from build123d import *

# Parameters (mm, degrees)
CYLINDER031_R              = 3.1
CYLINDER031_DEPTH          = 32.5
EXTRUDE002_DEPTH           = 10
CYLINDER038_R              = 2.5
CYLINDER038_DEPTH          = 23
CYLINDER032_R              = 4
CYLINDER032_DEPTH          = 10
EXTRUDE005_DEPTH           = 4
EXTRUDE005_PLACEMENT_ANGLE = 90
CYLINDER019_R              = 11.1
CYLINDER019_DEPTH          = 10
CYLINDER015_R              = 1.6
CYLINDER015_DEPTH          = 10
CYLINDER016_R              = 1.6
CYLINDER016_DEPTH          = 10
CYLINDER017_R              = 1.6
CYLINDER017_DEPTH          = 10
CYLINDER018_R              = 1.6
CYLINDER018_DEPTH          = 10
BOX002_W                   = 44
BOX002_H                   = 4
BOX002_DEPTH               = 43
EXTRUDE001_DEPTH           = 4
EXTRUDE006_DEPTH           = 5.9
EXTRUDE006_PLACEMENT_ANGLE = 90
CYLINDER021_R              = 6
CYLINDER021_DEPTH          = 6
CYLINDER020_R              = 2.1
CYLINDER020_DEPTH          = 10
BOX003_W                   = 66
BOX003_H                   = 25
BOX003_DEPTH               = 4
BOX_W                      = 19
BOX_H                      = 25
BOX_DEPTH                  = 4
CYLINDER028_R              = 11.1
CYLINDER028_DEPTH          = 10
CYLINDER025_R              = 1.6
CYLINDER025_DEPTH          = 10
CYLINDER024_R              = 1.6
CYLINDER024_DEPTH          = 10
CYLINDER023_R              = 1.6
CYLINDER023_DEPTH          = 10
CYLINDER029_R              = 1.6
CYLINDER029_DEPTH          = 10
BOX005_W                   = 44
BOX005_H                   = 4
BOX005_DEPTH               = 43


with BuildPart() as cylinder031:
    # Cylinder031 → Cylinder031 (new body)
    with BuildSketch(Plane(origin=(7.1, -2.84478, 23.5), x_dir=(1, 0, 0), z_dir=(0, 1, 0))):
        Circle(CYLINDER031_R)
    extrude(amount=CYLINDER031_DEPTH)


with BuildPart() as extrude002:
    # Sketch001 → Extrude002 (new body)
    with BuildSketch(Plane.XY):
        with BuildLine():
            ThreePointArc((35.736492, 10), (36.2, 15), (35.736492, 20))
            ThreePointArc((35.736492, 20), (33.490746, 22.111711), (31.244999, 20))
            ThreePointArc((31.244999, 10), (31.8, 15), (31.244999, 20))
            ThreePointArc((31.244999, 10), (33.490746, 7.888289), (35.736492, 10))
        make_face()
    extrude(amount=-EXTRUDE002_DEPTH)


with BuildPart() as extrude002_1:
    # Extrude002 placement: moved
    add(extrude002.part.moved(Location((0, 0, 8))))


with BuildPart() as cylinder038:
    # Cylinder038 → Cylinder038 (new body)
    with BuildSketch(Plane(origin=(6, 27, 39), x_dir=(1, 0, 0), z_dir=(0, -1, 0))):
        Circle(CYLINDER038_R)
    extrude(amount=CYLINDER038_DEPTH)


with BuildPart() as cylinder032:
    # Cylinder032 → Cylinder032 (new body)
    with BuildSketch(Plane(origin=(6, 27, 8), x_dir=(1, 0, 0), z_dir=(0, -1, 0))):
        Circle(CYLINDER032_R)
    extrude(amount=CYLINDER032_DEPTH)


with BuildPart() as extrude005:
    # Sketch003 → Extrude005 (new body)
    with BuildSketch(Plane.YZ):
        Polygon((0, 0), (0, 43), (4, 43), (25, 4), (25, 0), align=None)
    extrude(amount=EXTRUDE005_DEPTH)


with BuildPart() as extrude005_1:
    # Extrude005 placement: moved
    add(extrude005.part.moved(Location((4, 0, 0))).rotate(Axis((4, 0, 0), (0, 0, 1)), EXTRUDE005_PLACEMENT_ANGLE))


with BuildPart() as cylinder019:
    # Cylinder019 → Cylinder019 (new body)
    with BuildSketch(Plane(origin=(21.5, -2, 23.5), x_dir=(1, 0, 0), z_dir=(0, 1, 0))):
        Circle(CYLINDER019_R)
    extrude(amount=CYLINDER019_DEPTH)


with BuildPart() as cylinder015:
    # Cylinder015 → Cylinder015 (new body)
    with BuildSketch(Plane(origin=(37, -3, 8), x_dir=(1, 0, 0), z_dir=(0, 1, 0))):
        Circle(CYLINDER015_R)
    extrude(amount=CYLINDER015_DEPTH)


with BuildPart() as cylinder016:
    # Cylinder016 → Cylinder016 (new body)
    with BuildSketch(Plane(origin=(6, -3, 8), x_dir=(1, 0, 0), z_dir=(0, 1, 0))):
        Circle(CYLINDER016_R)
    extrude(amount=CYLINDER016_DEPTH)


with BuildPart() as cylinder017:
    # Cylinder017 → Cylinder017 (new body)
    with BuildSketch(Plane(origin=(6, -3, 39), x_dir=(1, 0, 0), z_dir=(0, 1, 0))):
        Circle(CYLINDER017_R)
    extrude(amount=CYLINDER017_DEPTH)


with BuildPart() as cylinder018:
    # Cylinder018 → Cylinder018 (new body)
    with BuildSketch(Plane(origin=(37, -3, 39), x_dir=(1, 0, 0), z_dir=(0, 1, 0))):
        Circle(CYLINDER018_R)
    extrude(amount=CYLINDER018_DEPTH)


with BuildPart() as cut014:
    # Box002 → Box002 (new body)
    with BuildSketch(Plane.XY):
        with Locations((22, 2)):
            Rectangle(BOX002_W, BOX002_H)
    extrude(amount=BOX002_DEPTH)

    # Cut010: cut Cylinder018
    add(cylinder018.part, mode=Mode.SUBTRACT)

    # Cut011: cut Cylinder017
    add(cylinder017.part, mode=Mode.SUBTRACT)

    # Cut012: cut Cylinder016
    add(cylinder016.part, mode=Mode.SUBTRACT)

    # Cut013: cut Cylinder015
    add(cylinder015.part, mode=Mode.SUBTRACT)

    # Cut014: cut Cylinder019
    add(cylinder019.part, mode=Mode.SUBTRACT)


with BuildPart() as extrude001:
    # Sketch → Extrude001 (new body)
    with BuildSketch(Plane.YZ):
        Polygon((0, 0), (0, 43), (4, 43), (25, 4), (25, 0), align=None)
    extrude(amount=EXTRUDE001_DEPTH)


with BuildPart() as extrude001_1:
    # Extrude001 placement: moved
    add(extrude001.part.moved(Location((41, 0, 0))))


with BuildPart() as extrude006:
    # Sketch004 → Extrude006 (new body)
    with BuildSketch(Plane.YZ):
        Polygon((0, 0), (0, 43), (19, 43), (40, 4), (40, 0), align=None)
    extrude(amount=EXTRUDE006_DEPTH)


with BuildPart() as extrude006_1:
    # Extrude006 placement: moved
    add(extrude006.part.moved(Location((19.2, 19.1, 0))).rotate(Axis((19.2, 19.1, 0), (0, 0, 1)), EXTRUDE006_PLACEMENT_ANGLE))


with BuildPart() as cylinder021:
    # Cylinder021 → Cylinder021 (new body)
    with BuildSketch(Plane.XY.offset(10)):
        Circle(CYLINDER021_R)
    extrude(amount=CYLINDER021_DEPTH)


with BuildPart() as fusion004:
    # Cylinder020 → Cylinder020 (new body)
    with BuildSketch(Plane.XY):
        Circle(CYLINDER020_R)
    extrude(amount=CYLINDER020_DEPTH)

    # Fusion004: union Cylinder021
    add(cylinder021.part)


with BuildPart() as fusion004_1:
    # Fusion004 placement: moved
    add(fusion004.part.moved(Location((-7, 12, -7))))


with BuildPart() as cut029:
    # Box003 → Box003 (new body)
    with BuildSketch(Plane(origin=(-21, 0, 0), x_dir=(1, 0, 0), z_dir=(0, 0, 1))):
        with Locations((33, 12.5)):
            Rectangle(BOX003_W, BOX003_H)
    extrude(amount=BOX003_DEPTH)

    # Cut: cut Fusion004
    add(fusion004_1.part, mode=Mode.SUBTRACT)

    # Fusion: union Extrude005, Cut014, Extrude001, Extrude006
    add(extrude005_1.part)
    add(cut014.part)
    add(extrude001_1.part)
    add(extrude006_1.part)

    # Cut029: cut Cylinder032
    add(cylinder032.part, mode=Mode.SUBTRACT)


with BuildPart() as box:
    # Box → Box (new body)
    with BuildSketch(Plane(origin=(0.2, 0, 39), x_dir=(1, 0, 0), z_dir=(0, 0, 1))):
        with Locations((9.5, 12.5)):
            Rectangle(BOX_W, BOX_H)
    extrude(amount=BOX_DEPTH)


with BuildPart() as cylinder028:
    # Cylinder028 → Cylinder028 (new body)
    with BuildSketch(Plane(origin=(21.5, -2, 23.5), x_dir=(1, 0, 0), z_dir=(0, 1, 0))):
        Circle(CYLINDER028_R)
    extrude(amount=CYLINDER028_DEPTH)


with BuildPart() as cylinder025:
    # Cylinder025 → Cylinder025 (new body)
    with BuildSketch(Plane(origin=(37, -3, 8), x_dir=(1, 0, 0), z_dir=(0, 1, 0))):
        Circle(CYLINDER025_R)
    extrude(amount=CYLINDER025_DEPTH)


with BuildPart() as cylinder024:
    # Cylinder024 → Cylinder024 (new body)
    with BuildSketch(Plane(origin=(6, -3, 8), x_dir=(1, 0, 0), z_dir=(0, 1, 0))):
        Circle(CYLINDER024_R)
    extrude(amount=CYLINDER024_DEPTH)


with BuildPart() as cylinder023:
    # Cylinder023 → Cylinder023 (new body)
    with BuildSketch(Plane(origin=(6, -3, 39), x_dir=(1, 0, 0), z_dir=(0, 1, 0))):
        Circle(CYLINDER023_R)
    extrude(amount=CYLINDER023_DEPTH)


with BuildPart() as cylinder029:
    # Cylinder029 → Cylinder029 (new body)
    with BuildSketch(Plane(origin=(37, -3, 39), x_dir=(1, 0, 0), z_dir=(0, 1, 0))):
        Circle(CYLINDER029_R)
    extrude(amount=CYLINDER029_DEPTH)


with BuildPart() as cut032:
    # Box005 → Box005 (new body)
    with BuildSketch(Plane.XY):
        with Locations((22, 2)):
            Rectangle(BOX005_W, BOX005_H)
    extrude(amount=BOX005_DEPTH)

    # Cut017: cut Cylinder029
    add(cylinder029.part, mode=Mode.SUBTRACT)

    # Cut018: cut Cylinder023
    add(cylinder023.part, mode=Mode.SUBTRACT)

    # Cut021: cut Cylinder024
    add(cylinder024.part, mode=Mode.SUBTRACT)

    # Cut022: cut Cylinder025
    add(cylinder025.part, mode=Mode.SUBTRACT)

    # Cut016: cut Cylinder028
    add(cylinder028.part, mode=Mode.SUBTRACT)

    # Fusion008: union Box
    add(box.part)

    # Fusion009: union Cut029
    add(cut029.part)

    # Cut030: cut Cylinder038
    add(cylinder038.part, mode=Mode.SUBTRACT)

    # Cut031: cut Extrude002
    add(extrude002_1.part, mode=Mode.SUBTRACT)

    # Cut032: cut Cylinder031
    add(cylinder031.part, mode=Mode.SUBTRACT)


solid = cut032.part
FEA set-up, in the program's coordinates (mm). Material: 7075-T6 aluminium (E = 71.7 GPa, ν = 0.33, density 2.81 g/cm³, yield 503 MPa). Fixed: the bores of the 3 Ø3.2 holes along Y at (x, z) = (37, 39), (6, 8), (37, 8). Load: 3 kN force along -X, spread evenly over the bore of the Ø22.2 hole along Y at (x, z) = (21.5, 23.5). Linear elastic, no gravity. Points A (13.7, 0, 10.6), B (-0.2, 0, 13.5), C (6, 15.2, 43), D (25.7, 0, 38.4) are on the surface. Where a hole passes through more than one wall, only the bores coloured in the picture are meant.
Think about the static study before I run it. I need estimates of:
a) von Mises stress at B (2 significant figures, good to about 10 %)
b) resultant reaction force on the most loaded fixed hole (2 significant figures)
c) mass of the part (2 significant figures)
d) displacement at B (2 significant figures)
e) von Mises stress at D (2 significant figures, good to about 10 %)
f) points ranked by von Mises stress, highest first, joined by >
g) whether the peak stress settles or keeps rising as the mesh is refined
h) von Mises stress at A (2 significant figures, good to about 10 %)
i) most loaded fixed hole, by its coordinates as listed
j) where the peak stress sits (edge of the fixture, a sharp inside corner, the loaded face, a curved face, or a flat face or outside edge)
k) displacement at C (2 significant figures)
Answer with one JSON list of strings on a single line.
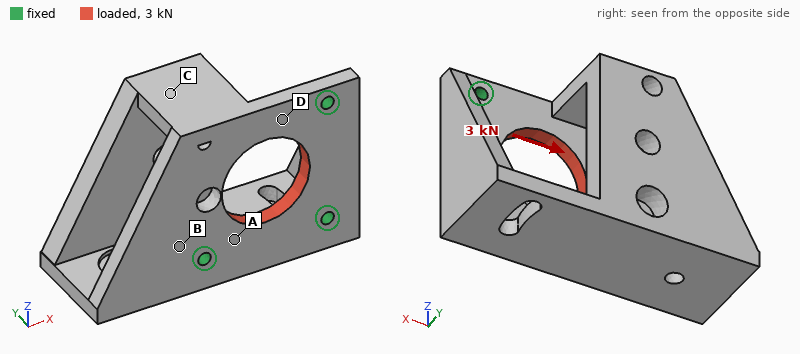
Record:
["8.7 MPa", "1.3 kN", "62 g", "2.9 µm", "23 MPa", "D > A > B > C", "keeps rising", "17 MPa", "(37, 39)", "a sharp inside corner", "6.5 µm"]
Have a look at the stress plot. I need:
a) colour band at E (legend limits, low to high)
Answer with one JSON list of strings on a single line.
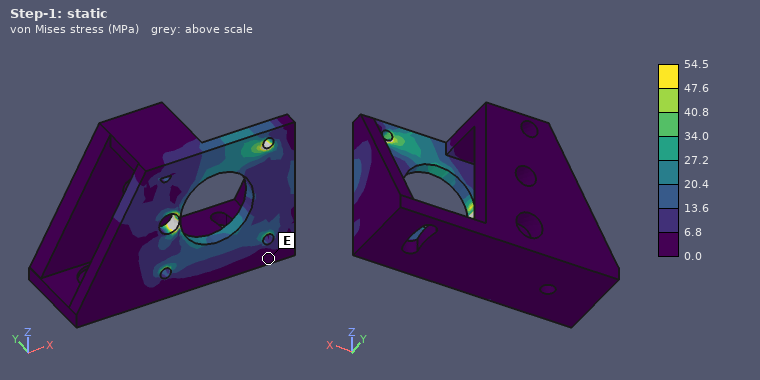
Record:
["0.0 to 6.8 MPa"]
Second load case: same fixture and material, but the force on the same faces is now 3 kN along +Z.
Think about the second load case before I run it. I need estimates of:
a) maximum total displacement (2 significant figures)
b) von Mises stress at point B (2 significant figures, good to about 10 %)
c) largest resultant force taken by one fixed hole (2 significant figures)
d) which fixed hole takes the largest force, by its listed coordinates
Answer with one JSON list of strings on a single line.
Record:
["15 µm", "11 MPa", "1.3 kN", "(6, 8)"]
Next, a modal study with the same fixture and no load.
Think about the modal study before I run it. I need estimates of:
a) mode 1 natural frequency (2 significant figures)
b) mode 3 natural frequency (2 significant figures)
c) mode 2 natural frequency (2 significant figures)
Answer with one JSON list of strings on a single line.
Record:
["2700 Hz", "5800 Hz", "4100 Hz"]
